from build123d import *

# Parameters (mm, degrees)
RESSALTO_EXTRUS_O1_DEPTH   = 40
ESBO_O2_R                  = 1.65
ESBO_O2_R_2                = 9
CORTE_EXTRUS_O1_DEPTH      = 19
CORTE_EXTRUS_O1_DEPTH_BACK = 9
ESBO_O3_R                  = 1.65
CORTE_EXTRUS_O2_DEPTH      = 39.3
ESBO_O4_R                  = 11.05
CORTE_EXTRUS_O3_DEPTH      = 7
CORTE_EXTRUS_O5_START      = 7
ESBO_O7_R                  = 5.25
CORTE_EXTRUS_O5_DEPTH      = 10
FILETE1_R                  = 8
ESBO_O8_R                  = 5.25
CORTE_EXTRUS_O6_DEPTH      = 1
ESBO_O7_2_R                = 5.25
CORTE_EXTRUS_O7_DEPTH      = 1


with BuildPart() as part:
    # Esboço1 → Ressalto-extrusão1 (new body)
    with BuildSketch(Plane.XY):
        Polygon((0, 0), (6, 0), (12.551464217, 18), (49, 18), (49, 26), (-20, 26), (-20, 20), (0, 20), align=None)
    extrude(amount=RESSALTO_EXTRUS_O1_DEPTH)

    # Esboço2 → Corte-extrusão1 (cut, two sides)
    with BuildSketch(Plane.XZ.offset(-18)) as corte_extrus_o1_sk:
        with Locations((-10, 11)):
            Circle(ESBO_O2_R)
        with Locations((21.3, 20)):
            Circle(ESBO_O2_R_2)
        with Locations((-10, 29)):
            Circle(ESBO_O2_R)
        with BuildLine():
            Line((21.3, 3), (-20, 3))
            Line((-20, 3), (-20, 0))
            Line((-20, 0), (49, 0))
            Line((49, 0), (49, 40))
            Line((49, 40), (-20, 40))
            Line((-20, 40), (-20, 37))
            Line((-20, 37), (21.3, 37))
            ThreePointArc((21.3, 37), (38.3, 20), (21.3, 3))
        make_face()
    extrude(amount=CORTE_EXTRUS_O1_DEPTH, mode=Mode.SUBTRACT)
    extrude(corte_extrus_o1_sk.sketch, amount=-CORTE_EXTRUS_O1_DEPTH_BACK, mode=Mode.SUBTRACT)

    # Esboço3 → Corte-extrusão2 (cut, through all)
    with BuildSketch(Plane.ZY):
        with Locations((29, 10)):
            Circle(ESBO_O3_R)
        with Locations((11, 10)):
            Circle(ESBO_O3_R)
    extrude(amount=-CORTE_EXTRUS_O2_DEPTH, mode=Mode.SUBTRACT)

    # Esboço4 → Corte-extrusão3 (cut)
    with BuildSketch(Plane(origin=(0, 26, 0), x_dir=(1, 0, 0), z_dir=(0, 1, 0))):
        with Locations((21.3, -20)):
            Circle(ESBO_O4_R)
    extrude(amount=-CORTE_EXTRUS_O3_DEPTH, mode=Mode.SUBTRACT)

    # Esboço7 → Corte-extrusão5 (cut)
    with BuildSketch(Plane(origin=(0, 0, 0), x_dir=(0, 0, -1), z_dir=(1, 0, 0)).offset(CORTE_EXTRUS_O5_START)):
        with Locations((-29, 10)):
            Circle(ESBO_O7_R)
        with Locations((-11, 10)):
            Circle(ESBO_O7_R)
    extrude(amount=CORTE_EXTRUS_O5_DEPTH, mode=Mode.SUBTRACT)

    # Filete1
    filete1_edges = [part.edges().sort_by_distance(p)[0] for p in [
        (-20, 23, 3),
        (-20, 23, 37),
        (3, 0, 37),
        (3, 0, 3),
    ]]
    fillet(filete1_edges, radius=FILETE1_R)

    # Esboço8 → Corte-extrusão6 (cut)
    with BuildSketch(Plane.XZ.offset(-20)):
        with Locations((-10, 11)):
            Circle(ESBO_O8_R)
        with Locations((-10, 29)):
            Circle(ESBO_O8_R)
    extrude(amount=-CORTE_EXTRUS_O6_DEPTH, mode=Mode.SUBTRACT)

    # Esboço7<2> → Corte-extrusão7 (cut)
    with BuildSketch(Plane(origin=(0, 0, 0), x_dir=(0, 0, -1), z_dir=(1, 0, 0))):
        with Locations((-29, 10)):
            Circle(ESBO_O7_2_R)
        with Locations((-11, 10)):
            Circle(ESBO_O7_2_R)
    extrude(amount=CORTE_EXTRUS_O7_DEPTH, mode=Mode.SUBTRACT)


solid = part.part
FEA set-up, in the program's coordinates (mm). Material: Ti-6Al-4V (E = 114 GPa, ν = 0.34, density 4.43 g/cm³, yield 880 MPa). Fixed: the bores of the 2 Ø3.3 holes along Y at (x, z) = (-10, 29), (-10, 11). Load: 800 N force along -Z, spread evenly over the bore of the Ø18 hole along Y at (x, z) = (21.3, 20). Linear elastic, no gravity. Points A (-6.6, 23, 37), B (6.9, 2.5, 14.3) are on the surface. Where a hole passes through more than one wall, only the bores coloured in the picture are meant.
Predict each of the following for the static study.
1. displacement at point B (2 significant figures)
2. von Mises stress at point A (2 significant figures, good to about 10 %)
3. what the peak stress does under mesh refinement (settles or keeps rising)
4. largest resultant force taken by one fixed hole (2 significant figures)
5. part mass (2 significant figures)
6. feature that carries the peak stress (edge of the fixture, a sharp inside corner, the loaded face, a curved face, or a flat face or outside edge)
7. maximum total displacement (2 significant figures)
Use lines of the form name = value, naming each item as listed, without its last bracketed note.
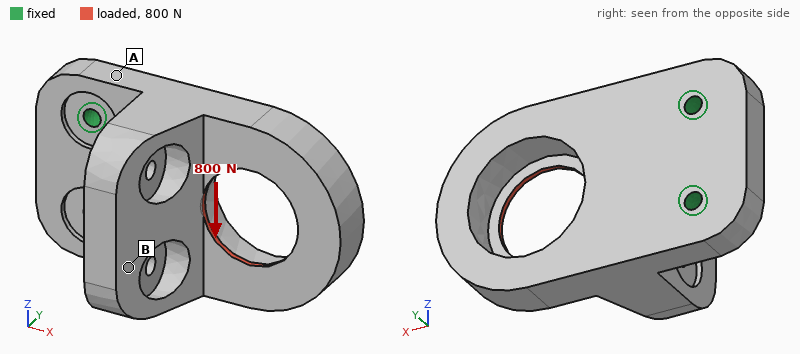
displacement at point B = 6.6 µm
von Mises stress at point A = 13 MPa
what the peak stress does under mesh refinement = keeps rising
largest resultant force taken by one fixed hole = 1.3 kN
part mass = 66 g
feature that carries the peak stress = edge of the fixture
maximum total displacement = 21 µm
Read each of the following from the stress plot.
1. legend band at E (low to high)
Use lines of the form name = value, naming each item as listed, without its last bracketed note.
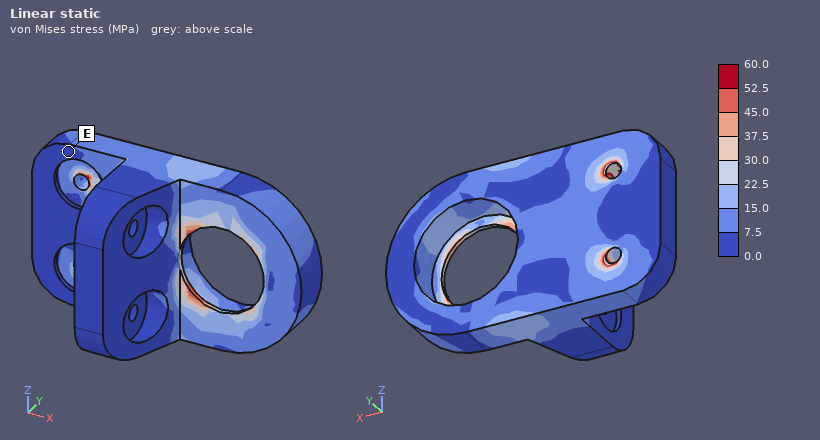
legend band at E = 0.0 to 7.5 MPa
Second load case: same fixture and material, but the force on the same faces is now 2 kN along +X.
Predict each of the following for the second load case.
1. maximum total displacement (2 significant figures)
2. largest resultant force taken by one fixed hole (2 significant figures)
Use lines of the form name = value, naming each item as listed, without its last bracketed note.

maximum total displacement = 0.11 mm
largest resultant force taken by one fixed hole = 1.0 kN
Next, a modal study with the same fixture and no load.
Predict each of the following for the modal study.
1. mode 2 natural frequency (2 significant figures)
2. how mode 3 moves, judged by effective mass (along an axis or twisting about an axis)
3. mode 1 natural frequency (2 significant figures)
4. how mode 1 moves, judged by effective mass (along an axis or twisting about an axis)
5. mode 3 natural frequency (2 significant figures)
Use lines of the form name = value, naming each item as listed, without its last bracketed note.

mode 2 natural frequency = 6400 Hz
how mode 3 moves, judged by effective mass = along Z
mode 1 natural frequency = 2100 Hz
how mode 1 moves, judged by effective mass = along Y
mode 3 natural frequency = 7400 Hz
